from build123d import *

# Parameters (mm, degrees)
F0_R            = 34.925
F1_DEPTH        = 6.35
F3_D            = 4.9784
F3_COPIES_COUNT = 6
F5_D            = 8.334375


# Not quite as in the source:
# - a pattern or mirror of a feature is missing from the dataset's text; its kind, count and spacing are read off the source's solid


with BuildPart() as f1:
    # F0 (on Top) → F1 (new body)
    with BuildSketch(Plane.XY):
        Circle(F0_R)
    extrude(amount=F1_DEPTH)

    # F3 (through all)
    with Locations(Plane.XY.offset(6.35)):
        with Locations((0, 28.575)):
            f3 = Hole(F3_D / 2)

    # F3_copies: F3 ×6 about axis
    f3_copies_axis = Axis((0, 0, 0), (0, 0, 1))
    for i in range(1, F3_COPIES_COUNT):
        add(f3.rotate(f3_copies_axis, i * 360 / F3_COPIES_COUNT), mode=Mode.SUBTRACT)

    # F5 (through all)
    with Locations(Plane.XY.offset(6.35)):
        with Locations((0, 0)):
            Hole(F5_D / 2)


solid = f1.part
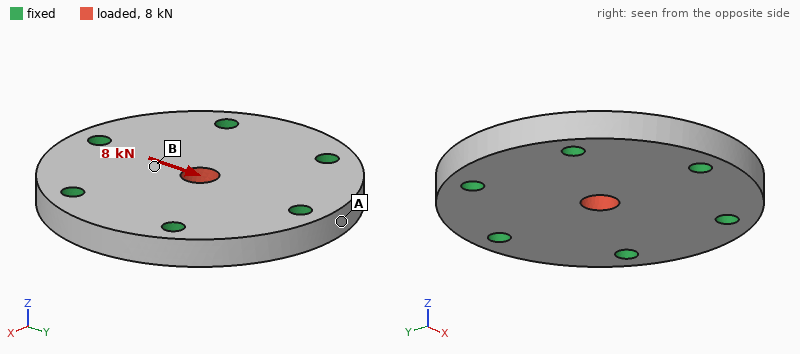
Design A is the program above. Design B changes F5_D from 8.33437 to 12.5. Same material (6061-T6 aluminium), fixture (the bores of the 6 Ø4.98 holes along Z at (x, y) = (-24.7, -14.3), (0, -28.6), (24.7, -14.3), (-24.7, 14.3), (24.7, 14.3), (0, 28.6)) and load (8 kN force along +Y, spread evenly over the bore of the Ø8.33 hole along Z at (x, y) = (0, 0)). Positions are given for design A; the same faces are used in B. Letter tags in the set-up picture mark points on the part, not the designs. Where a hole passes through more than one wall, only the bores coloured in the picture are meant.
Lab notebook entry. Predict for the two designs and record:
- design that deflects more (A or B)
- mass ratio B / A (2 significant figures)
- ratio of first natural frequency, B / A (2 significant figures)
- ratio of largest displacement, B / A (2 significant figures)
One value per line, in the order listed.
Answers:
A
0.98
1.0
0.79
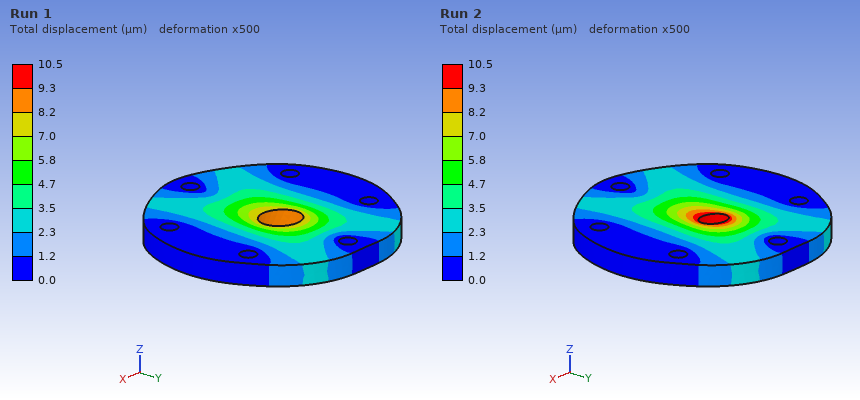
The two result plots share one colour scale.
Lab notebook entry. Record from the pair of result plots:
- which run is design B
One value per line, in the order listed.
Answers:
Run 1
